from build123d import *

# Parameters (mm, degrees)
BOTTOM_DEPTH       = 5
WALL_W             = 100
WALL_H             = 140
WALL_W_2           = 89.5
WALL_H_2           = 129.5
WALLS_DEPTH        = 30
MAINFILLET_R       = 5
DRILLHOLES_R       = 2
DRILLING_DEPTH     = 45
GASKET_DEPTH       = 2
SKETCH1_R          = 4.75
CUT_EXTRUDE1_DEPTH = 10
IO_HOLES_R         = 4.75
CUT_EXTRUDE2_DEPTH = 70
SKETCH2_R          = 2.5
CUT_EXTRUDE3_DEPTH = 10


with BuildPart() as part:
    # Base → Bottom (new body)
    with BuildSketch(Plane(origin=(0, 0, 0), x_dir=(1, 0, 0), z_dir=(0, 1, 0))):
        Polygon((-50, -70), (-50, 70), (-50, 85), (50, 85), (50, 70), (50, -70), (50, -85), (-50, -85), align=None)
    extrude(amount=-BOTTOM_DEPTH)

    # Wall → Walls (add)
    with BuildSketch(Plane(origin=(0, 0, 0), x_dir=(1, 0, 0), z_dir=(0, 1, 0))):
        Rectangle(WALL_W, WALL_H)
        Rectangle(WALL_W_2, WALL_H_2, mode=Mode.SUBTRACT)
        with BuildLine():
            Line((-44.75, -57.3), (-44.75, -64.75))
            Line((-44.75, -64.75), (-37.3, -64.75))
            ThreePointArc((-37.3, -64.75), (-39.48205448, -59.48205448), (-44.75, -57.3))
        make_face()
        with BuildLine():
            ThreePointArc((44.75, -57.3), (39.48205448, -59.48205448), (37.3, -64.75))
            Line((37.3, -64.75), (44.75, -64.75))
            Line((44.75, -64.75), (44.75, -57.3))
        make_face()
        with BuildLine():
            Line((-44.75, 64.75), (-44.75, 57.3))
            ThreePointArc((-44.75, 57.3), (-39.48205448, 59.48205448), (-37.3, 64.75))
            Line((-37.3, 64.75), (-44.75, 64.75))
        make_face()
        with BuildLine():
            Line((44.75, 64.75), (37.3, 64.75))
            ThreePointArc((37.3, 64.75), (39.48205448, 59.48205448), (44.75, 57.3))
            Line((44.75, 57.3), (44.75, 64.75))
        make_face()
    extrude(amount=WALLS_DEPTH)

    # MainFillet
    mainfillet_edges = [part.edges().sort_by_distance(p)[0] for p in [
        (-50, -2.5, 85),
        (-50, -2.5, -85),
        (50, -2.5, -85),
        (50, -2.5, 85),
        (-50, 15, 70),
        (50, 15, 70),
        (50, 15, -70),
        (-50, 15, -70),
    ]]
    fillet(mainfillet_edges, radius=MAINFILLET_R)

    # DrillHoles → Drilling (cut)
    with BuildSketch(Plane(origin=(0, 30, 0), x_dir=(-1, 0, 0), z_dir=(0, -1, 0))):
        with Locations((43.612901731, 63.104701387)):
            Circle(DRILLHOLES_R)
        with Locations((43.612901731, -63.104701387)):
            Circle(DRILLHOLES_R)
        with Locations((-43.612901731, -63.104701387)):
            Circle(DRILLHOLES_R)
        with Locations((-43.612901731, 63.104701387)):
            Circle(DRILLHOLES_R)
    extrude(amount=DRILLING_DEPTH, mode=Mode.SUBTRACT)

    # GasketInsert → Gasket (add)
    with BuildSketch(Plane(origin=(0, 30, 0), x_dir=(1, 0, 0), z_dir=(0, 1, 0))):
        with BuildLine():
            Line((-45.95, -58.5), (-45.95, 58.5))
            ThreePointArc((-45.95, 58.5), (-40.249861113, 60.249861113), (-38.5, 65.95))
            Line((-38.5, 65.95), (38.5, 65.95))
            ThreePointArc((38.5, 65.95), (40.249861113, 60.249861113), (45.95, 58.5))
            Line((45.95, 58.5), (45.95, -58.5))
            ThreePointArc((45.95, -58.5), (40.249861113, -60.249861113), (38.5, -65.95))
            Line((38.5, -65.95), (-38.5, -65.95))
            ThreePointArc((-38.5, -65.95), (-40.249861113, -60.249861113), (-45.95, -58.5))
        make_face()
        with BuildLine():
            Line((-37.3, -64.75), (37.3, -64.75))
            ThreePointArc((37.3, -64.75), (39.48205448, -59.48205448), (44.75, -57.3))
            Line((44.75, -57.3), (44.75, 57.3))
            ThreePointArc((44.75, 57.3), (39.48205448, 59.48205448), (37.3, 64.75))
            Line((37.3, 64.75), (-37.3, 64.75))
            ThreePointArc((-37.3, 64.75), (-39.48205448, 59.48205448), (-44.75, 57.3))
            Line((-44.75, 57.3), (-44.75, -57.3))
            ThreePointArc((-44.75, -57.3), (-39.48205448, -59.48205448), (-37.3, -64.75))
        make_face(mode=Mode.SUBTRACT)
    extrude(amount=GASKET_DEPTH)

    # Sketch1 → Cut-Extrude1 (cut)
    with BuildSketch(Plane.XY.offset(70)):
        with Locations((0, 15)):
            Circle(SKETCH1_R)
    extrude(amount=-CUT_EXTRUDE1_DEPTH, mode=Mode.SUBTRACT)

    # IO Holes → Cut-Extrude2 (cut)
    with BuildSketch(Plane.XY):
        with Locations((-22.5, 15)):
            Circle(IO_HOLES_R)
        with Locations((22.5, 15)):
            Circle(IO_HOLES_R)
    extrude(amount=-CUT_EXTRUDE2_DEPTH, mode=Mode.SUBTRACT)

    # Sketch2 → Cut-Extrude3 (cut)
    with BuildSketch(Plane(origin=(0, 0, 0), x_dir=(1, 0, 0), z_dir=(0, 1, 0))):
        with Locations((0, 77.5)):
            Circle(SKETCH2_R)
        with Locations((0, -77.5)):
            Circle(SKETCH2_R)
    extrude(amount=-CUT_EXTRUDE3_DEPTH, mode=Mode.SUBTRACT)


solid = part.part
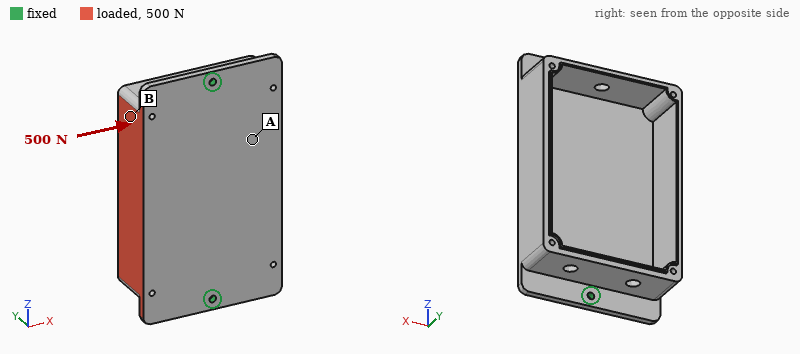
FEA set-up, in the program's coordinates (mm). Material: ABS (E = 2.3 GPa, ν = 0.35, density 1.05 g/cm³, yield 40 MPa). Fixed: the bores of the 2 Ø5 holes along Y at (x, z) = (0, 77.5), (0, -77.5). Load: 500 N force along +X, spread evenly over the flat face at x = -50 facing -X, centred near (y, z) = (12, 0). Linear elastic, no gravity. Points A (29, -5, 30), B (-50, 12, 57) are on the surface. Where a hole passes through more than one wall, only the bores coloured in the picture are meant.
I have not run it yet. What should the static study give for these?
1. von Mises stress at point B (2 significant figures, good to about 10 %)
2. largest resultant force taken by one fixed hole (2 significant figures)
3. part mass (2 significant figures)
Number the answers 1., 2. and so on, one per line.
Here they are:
1. 4.4 MPa
2. 250 N
3. 170 g
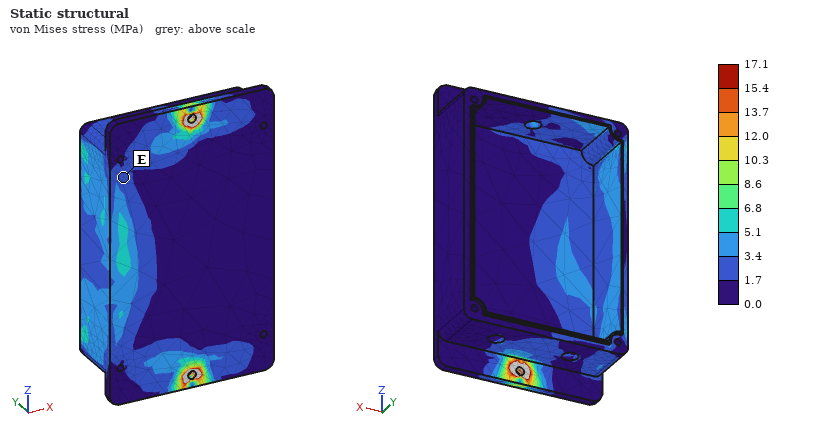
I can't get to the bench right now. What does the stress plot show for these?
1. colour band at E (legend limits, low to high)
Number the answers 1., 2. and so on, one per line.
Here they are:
1. 1.7 to 3.4 MPa
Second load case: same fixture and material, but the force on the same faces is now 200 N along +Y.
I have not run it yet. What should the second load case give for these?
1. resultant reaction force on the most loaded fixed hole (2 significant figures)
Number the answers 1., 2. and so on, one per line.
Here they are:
1. 110 N
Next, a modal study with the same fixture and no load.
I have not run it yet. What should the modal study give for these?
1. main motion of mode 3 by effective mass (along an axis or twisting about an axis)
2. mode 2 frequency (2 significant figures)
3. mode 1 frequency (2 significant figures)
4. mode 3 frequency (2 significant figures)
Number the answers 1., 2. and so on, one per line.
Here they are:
1. along Y
2. 380 Hz
3. 170 Hz
4. 540 Hz
